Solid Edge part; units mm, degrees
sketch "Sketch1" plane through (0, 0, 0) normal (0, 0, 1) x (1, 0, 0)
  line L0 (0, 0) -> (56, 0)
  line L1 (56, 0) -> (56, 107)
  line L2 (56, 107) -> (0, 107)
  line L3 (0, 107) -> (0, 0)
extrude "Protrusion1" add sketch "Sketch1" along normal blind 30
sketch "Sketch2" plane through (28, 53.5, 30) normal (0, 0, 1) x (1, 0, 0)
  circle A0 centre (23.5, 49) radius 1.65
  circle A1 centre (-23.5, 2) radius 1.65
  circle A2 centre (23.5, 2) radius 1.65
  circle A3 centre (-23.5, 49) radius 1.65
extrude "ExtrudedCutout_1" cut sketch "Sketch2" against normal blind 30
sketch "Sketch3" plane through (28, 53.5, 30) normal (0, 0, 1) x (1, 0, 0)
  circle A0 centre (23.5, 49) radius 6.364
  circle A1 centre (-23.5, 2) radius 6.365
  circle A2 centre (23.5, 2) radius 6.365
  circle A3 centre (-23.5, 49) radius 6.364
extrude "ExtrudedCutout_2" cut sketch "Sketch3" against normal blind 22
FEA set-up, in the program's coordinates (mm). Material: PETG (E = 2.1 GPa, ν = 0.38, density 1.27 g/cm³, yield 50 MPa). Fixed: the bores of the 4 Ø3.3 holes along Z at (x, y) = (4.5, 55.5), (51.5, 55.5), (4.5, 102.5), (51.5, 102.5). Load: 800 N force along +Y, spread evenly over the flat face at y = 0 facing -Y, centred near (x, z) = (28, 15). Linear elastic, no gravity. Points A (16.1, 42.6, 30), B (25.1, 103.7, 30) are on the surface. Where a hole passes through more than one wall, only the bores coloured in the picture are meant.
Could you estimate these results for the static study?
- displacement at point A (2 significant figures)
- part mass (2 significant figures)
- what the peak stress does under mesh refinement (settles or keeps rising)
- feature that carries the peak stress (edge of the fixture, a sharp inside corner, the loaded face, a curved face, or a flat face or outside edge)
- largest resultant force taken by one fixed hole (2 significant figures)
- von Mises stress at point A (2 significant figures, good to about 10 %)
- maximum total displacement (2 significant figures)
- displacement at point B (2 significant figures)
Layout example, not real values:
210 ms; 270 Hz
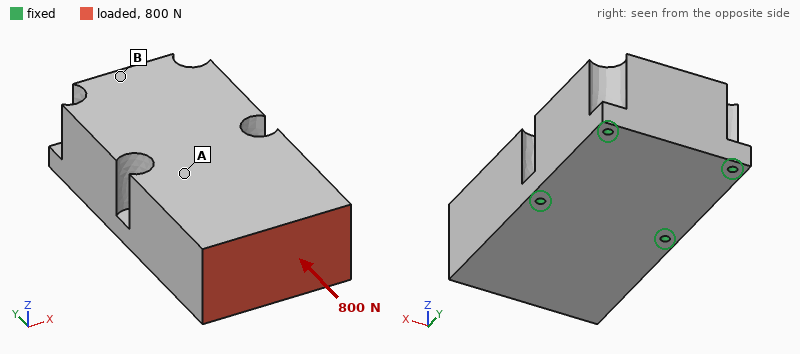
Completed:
43 µm; 220 g; keeps rising; edge of the fixture; 280 N; 0.89 MPa; 82 µm; 26 µm
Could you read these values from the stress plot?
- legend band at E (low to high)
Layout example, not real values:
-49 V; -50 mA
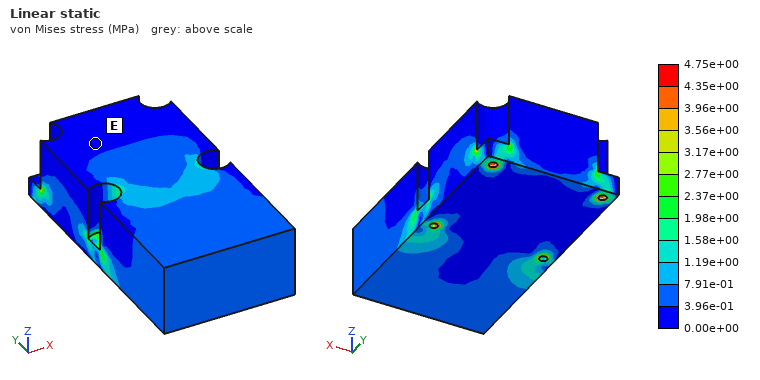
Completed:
0.00e+00 to 3.96e-01 MPa
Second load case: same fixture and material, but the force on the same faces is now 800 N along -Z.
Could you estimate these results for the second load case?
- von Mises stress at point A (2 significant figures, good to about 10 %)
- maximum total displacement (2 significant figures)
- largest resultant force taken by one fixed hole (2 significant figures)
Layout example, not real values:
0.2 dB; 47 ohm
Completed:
5.6 MPa; 0.67 mm; 940 N
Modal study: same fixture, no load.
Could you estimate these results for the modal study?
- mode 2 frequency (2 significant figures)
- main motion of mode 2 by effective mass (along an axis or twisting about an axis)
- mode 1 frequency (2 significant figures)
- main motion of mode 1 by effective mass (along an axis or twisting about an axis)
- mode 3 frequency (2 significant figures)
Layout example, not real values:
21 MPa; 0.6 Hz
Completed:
1500 Hz; along X; 840 Hz; along Z; 2000 Hz
